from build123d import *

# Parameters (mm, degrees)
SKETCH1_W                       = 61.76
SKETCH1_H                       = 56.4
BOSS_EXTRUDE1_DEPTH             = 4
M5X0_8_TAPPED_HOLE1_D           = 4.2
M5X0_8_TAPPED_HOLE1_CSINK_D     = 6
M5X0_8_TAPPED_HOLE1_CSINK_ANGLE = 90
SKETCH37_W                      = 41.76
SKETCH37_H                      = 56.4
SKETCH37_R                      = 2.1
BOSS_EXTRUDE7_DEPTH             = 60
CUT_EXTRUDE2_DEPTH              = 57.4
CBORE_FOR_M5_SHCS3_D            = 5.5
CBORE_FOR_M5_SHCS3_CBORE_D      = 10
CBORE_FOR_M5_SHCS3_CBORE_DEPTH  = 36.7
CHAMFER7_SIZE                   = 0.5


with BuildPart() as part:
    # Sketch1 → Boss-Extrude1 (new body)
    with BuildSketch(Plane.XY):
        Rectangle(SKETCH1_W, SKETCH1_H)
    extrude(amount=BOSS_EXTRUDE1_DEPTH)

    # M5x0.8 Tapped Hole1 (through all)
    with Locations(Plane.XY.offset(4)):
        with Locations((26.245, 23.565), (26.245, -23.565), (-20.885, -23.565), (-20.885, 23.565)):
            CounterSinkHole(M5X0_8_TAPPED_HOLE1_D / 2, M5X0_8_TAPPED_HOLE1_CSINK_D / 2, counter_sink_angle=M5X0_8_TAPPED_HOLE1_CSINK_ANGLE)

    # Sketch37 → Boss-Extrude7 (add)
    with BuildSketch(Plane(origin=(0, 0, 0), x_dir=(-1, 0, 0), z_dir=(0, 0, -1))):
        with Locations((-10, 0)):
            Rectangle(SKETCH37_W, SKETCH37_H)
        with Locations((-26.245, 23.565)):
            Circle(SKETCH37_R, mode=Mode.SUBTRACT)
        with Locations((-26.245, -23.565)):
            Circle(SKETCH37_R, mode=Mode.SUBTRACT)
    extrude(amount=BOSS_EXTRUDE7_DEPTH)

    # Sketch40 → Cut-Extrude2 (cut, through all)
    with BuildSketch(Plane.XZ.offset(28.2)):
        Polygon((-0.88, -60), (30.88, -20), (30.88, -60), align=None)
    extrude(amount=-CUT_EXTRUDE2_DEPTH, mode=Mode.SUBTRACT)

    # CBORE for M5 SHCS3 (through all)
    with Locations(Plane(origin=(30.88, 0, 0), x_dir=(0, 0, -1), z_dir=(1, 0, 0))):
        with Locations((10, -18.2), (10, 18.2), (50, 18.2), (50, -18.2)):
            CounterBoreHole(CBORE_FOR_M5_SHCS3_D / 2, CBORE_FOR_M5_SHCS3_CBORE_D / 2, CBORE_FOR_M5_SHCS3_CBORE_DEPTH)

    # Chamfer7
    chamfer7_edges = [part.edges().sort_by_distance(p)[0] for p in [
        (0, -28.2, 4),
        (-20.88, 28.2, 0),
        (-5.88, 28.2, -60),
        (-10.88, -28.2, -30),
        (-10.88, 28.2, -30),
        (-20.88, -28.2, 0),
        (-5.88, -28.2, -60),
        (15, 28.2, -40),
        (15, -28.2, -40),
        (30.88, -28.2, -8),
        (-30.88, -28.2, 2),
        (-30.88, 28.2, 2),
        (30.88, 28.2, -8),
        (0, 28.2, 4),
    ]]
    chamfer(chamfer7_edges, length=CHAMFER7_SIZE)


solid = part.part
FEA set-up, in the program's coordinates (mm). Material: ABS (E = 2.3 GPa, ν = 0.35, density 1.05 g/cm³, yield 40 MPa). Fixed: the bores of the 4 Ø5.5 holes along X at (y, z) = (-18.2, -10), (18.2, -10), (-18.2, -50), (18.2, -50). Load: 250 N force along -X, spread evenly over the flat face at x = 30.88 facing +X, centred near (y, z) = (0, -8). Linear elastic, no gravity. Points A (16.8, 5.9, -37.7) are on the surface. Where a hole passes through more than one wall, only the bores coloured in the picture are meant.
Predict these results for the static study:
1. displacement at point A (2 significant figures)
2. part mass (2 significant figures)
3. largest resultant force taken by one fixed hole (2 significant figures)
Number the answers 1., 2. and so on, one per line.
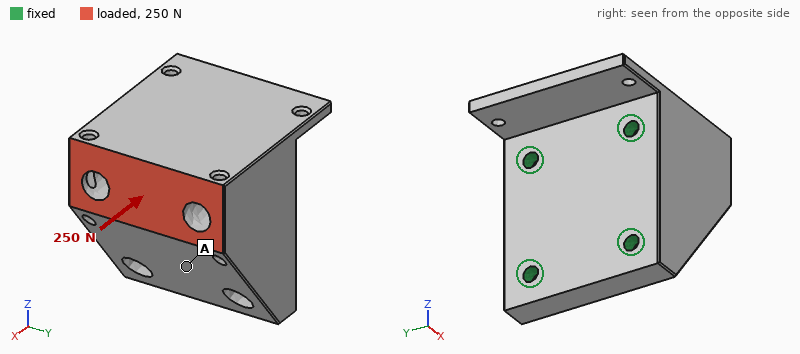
1. 5.5 µm
2. 120 g
3. 130 N
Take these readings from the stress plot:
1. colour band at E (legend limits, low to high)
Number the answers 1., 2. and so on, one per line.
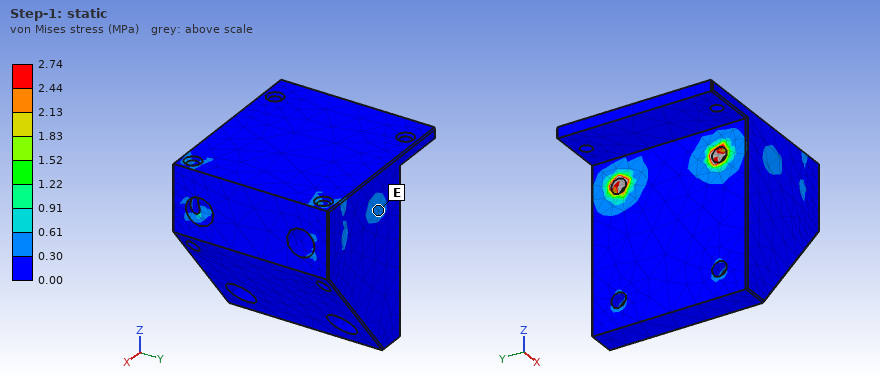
1. 0.30 to 0.61 MPa
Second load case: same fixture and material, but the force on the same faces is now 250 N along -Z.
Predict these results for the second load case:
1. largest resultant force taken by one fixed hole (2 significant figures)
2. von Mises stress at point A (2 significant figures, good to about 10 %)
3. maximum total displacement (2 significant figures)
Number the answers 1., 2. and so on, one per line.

1. 150 N
2. 0.49 MPa
3. 36 µm
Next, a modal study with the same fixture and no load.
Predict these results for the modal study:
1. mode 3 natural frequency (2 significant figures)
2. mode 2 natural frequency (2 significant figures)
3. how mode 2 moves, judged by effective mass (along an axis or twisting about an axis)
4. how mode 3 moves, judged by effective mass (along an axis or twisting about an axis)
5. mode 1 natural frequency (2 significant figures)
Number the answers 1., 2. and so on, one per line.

1. 2600 Hz
2. 2500 Hz
3. along Y
4. along Z
5. 1900 Hz
